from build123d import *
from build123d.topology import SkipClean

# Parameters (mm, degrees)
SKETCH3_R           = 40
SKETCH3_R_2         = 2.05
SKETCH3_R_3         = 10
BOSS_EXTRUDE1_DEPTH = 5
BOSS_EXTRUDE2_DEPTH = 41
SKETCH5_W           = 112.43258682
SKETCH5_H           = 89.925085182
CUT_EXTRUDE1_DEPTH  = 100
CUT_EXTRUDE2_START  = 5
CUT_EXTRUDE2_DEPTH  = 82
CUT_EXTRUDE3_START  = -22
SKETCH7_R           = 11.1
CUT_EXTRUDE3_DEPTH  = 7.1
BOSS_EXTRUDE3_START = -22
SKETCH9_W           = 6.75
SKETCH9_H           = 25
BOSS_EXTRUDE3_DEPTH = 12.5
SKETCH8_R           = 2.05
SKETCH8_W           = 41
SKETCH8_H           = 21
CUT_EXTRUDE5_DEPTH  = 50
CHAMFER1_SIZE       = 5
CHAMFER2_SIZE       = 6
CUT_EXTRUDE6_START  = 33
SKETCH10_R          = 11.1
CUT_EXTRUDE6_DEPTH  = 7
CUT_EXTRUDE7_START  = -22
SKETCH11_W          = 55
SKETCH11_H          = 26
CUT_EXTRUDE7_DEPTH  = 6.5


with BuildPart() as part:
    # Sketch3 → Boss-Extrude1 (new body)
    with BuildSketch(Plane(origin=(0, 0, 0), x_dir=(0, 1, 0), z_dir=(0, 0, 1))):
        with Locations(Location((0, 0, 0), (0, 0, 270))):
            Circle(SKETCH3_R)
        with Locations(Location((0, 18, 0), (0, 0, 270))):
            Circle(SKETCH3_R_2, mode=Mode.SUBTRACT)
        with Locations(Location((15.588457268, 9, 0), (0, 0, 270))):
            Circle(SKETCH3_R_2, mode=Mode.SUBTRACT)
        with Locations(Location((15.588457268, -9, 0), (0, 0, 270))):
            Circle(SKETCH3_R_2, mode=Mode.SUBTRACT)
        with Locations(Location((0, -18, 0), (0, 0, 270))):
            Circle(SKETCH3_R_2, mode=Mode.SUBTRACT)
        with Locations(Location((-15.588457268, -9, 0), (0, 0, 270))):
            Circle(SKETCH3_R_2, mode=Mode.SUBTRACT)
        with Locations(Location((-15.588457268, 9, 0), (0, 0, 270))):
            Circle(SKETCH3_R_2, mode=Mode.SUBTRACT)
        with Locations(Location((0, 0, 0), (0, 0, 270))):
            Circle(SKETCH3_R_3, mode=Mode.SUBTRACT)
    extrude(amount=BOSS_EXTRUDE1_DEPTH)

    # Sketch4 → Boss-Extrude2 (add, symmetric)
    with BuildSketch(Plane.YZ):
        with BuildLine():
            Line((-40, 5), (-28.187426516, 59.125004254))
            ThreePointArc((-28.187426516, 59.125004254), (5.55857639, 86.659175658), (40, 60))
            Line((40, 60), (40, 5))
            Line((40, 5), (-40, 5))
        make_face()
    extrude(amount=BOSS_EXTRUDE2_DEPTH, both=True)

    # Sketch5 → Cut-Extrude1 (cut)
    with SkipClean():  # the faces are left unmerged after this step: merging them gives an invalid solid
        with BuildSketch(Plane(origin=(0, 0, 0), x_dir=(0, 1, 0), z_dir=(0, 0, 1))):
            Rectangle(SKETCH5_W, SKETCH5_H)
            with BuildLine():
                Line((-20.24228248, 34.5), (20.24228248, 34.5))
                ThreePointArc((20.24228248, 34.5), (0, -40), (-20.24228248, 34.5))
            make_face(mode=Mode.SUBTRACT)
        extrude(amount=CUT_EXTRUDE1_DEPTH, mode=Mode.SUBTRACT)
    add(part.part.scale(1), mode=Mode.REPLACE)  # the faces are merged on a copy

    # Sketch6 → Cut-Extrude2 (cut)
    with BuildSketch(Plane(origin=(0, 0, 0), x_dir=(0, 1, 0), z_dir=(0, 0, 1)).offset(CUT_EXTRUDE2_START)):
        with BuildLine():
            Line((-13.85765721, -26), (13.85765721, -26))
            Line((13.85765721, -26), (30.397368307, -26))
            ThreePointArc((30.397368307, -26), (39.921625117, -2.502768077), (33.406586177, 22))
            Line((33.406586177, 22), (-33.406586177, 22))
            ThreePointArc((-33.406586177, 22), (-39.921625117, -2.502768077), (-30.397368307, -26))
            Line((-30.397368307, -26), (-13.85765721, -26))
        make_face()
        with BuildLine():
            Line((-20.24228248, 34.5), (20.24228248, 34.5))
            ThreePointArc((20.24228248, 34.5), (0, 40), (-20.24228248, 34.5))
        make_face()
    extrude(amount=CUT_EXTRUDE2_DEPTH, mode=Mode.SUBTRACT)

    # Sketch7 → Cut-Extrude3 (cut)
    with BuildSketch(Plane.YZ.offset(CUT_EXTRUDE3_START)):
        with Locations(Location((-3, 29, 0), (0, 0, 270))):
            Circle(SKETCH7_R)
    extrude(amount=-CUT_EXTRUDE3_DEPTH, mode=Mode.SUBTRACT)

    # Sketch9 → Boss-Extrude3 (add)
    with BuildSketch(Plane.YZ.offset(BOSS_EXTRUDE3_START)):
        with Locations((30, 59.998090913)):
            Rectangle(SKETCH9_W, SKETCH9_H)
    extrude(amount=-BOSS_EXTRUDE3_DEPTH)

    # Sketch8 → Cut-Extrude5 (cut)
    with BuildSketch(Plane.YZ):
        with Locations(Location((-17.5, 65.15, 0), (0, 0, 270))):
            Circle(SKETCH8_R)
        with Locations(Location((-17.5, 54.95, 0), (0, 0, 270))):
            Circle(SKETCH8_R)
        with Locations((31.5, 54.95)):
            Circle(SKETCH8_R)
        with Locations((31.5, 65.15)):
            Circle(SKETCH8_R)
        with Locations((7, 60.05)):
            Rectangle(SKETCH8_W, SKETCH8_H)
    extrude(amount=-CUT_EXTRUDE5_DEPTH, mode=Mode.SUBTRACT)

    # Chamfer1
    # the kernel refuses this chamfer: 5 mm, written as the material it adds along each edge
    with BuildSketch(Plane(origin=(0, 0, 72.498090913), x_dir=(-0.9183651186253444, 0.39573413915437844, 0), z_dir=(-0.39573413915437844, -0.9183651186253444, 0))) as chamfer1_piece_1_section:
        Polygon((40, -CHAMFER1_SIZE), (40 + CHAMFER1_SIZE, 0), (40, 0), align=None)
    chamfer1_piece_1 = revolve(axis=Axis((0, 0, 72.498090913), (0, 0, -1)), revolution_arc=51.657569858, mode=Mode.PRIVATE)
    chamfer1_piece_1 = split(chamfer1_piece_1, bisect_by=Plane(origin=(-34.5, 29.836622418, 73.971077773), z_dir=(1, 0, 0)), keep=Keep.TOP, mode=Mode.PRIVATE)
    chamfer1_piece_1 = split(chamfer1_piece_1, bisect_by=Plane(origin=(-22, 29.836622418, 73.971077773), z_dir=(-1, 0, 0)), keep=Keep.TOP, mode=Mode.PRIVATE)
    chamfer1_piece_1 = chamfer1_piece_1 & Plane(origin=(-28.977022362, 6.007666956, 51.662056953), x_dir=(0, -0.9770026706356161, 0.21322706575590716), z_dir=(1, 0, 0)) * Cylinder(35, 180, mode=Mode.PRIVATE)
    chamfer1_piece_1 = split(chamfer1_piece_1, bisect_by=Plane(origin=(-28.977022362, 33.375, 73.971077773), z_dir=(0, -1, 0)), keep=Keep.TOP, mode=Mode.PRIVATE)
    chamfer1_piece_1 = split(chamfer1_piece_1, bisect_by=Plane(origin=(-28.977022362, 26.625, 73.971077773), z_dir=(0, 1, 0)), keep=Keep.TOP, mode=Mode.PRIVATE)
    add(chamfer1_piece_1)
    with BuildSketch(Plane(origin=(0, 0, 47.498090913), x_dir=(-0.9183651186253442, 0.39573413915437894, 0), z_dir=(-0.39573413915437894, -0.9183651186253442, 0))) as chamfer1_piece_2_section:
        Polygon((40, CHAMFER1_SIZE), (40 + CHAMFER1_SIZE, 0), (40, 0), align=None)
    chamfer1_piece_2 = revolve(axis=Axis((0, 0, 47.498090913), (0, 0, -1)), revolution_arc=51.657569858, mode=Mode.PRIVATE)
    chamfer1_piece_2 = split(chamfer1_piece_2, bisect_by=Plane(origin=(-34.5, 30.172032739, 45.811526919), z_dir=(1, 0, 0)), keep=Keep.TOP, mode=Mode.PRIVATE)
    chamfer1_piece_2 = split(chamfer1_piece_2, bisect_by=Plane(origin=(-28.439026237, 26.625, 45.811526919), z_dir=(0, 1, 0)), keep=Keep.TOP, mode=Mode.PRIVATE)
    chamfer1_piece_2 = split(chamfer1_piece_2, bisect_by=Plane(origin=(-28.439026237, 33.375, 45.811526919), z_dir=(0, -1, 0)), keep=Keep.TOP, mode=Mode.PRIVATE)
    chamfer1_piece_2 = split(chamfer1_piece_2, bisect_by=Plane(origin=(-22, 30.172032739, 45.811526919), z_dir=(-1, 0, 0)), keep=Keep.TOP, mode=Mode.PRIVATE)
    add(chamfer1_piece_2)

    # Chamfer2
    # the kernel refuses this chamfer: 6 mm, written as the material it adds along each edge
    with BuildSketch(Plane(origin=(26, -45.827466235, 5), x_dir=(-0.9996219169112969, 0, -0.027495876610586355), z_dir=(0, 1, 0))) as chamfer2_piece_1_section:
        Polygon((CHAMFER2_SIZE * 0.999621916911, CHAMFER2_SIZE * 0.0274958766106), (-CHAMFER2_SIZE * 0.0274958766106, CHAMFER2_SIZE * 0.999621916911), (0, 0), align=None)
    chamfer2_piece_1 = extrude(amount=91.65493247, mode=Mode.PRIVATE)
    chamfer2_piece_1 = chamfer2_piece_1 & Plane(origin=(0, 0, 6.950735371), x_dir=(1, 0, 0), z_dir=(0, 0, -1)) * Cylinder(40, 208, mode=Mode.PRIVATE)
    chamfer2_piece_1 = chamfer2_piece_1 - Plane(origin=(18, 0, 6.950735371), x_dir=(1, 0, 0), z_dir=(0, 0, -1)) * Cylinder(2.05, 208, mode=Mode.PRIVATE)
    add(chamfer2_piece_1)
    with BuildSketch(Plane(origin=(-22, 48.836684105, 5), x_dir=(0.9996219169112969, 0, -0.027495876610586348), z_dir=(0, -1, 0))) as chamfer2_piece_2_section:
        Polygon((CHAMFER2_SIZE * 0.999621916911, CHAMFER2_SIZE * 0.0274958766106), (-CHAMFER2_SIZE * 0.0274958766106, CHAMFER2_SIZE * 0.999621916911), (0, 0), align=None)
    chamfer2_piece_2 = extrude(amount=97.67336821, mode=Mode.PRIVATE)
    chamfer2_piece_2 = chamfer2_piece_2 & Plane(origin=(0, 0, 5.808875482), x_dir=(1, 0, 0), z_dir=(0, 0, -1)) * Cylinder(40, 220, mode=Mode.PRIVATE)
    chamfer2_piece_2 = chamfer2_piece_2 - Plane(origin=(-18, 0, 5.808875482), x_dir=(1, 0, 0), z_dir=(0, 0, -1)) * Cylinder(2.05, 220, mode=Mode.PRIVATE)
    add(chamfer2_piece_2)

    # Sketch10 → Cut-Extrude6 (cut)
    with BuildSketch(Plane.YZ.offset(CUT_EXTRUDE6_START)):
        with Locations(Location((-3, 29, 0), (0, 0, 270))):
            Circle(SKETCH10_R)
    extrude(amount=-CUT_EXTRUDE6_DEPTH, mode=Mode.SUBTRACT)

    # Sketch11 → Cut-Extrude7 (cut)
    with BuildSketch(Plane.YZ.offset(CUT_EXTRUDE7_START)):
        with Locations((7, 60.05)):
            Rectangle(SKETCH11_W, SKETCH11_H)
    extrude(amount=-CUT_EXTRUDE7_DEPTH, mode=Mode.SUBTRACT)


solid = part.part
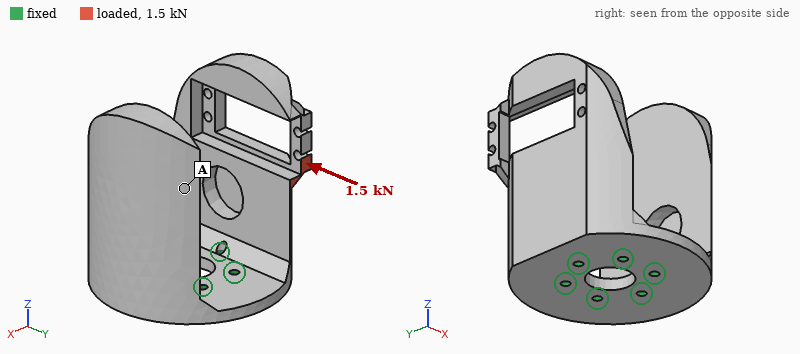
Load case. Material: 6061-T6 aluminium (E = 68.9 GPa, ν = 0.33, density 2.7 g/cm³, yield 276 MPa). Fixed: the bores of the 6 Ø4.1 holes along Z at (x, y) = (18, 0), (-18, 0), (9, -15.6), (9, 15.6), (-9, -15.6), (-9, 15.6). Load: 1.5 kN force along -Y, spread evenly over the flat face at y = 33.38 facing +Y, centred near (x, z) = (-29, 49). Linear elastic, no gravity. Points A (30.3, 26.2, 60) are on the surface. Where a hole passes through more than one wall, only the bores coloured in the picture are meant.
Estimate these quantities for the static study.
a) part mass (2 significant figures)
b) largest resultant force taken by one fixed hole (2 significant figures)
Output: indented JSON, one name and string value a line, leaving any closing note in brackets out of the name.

{
  "part mass": "280 g",
  "largest resultant force taken by one fixed hole": "1.8 kN"
}
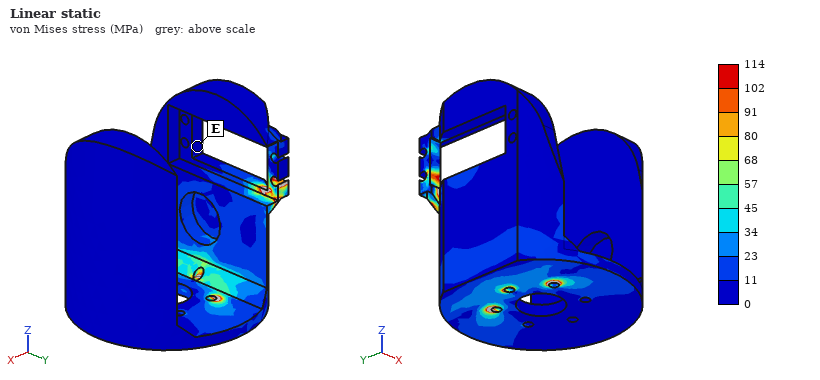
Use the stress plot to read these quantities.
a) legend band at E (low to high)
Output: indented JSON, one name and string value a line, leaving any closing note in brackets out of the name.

{
  "legend band at E": "0 to 11 MPa"
}
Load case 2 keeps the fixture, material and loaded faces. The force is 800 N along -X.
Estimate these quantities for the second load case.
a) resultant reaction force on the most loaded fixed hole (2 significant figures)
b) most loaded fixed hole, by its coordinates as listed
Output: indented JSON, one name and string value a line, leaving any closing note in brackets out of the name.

{
  "resultant reaction force on the most loaded fixed hole": "1.9 kN",
  "most loaded fixed hole, by its coordinates as listed": "(-18, 0)"
}
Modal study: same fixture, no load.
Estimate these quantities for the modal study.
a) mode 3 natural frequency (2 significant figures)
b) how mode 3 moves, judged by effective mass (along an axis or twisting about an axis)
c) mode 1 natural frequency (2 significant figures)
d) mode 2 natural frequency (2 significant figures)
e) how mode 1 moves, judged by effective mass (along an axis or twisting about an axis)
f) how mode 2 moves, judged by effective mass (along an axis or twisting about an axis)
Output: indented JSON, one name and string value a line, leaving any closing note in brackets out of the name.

{
  "mode 3 natural frequency": "1300 Hz",
  "how mode 3 moves, judged by effective mass": "along Y",
  "mode 1 natural frequency": "660 Hz",
  "mode 2 natural frequency": "900 Hz",
  "how mode 1 moves, judged by effective mass": "along X",
  "how mode 2 moves, judged by effective mass": "along X"
}
